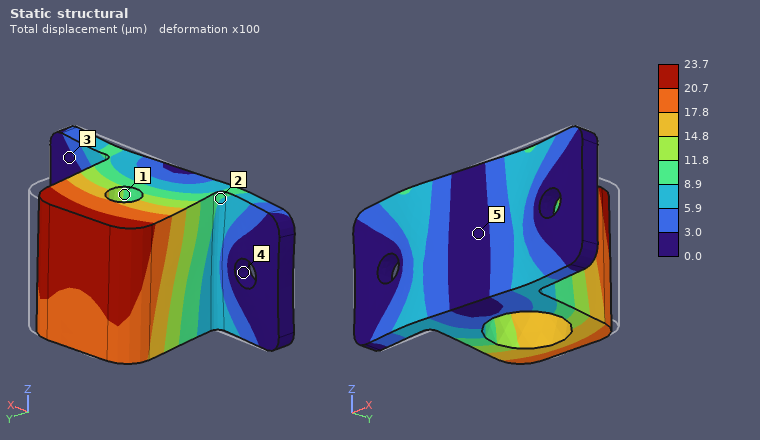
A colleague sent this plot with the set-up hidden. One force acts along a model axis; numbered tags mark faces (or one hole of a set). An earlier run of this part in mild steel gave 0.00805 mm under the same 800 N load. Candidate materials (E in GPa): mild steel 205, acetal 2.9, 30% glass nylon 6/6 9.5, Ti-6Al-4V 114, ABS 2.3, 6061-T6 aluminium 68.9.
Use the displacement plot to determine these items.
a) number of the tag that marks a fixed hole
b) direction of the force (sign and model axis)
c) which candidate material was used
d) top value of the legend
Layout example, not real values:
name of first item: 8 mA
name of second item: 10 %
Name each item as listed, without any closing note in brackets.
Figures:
number of the tag that marks a fixed hole: 4
direction of the force: -X
which candidate material was used: 6061-T6 aluminium
top value of the legend: 23.7 µm
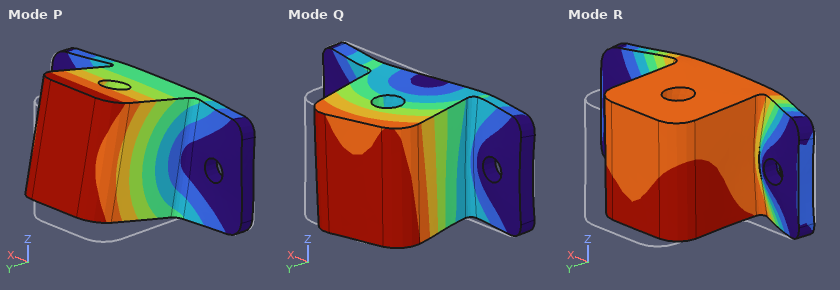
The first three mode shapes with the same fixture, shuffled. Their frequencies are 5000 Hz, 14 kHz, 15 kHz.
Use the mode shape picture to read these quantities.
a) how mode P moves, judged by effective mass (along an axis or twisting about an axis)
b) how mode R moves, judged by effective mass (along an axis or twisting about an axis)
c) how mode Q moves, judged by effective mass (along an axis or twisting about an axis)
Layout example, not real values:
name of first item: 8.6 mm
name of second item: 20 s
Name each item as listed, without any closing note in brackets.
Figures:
how mode P moves, judged by effective mass: along Z
how mode R moves, judged by effective mass: along Y
how mode Q moves, judged by effective mass: along X
